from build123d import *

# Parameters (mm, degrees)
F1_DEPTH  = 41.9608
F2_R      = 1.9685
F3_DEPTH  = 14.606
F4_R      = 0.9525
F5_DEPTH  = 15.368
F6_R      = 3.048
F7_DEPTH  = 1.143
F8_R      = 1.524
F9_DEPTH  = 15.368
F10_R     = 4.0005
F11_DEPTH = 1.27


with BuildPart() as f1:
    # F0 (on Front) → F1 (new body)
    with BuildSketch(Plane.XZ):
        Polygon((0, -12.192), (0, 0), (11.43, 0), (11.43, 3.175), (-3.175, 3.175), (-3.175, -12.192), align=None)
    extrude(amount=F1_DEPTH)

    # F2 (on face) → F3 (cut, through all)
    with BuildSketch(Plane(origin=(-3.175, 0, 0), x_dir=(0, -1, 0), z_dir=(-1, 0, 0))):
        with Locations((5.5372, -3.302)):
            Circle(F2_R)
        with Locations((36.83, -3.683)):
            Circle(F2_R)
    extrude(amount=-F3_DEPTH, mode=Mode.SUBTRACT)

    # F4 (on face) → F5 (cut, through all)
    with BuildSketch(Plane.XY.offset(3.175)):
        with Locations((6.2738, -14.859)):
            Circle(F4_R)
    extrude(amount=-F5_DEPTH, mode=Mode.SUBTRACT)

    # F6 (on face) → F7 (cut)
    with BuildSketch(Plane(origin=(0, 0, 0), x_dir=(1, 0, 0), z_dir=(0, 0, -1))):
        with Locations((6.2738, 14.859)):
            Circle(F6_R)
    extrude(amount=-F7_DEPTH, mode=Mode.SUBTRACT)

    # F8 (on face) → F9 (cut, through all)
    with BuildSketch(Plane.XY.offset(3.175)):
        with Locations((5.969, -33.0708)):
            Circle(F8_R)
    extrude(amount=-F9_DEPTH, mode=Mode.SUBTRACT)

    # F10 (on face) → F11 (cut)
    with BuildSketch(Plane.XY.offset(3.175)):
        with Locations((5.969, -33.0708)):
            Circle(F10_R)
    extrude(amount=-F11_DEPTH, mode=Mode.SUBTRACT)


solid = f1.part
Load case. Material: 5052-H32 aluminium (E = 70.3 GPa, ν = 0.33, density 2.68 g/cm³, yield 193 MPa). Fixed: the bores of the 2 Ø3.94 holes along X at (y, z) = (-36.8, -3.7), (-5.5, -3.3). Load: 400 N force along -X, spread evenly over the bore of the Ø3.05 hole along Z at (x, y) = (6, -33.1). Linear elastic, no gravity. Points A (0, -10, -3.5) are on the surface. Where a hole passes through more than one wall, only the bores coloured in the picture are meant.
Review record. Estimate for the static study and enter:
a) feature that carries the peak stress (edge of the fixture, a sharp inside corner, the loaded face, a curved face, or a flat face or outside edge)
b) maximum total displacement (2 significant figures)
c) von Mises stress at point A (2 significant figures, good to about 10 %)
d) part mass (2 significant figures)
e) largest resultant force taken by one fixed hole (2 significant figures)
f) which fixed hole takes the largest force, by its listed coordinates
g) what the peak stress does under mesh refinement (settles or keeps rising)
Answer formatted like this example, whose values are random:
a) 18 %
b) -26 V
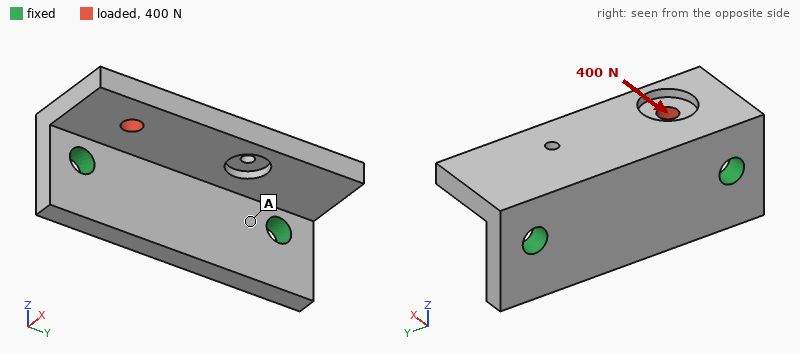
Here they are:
a) edge of the fixture
b) 11 µm
c) 5.9 MPa
d) 9.0 g
e) 360 N
f) (-36.8, -3.7)
g) keeps rising
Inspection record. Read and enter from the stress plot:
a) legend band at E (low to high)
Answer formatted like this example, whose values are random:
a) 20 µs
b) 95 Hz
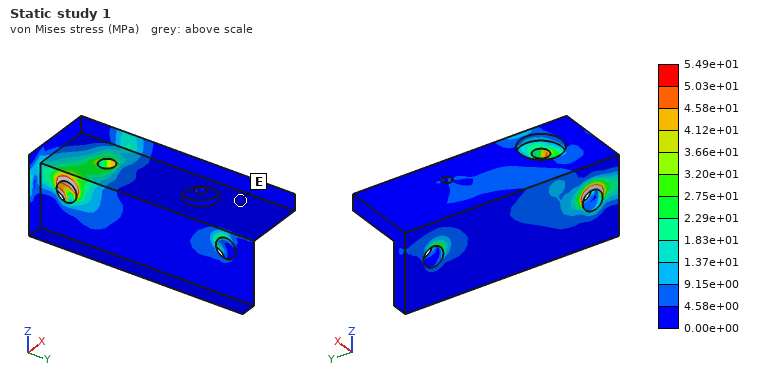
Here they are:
a) 0.00e+00 to 4.58e+00 MPa
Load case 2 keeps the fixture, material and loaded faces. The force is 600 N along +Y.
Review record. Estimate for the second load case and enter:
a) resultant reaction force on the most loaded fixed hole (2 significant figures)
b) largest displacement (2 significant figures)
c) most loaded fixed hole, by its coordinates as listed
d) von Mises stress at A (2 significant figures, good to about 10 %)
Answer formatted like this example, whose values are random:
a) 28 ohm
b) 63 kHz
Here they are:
a) 360 N
b) 12 µm
c) (-36.8, -3.7)
d) 8.8 MPa
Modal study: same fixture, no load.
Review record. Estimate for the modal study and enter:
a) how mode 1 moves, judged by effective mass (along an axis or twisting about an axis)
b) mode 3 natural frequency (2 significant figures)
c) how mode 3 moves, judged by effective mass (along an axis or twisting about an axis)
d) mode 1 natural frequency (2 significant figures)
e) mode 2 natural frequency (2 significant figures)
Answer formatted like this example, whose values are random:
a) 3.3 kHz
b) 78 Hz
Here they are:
a) along Z
b) 19 kHz
c) along X
d) 9400 Hz
e) 14 kHz
